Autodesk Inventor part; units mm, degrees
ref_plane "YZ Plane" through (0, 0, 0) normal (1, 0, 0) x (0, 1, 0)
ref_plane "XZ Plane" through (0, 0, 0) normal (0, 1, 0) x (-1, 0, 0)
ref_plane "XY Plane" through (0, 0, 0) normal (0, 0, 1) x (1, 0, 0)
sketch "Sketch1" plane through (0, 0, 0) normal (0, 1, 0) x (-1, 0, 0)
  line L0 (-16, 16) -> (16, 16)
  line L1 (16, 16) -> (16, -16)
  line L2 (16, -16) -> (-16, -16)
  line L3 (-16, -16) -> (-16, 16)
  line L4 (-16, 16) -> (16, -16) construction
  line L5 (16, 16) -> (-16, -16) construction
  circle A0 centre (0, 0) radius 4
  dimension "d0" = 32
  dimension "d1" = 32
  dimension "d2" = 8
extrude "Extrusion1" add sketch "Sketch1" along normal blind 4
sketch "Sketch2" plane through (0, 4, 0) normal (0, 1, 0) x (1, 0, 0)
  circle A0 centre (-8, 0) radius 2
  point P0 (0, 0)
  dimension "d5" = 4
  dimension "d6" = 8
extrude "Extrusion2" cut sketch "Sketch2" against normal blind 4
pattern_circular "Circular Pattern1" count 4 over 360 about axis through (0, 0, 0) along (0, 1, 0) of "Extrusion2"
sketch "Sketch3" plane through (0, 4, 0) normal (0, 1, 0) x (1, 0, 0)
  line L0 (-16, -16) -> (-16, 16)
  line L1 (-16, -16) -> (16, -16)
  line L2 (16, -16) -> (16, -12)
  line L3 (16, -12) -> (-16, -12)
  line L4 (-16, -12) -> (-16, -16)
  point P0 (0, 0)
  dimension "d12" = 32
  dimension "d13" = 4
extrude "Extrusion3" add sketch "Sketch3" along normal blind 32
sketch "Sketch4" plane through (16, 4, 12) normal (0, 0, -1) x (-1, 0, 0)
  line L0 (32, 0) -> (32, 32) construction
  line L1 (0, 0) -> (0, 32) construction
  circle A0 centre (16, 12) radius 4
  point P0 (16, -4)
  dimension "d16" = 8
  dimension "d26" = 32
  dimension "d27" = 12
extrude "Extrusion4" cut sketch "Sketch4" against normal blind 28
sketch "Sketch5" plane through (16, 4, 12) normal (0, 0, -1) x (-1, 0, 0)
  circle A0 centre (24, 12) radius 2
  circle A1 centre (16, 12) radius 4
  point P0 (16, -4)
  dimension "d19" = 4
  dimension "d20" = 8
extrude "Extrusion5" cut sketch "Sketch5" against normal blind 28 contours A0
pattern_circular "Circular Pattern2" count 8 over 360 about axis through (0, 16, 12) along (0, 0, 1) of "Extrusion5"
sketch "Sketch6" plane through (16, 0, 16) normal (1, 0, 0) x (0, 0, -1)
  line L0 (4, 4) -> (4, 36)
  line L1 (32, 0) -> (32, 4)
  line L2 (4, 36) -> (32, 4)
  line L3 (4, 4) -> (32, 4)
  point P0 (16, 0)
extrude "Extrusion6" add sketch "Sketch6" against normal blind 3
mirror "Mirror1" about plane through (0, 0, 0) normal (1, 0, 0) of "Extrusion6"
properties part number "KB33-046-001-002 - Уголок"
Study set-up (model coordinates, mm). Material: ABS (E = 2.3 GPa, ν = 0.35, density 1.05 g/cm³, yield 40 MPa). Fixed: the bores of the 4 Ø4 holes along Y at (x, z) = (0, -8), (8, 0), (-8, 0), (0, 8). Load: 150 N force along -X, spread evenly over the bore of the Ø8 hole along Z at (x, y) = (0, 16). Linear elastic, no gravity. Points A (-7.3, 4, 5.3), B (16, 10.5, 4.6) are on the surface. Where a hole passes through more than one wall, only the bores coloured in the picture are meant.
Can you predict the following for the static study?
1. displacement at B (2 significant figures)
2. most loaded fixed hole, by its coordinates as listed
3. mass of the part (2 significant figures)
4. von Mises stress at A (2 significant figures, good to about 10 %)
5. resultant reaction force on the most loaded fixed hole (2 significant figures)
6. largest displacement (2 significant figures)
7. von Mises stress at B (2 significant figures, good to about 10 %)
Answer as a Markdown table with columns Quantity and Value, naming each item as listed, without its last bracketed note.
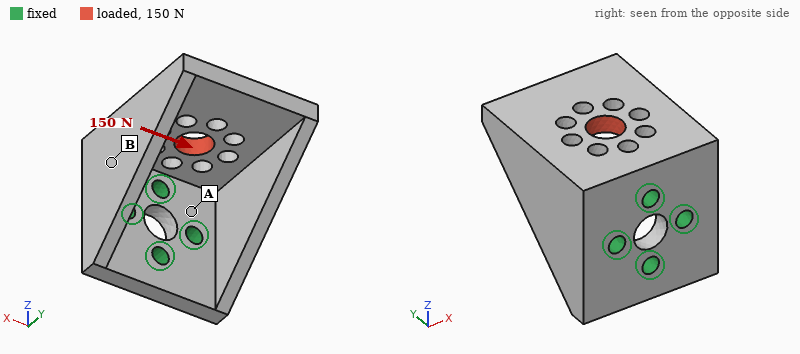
| Quantity | Value |
|---|---|
| displacement at B | 0.12 mm |
| most loaded fixed hole, by its coordinates as listed | (0, 8) |
| mass of the part | 10 g |
| von Mises stress at A | 5.4 MPa |
| resultant reaction force on the most loaded fixed hole | 140 N |
| largest displacement | 0.40 mm |
| von Mises stress at B | 2.3 MPa |
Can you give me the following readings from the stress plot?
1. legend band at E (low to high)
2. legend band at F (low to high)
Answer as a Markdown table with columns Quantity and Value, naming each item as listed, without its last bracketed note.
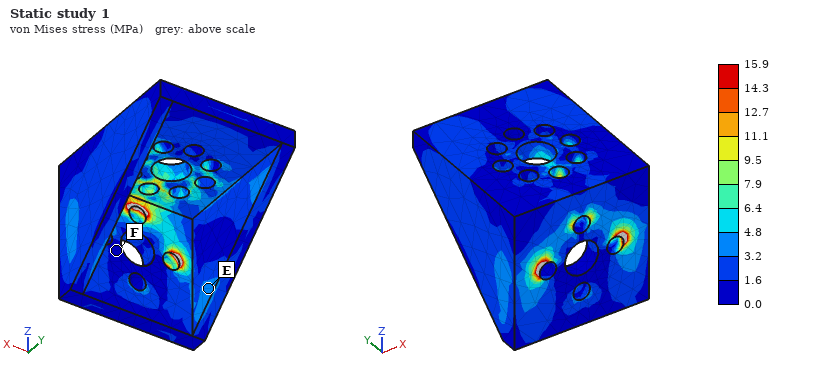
| Quantity | Value |
|---|---|
| legend band at E | 3.2 to 4.8 MPa |
| legend band at F | 0.0 to 1.6 MPa |
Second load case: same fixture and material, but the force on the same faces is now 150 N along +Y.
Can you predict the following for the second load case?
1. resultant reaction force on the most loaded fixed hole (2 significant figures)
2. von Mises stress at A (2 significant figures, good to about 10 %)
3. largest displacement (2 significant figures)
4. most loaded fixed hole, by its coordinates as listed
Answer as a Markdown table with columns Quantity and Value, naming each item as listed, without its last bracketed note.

| Quantity | Value |
|---|---|
| resultant reaction force on the most loaded fixed hole | 130 N |
| von Mises stress at A | 2.6 MPa |
| largest displacement | 0.14 mm |
| most loaded fixed hole, by its coordinates as listed | (0, 8) |
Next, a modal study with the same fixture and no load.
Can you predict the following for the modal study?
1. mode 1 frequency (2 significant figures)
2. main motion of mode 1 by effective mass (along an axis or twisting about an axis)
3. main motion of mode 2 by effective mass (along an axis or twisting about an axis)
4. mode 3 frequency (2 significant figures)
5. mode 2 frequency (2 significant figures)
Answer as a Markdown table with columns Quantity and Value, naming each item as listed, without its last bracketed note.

| Quantity | Value |
|---|---|
| mode 1 frequency | 1300 Hz |
| main motion of mode 1 by effective mass | along X |
| main motion of mode 2 by effective mass | along Z |
| mode 3 frequency | 3300 Hz |
| mode 2 frequency | 1700 Hz |
